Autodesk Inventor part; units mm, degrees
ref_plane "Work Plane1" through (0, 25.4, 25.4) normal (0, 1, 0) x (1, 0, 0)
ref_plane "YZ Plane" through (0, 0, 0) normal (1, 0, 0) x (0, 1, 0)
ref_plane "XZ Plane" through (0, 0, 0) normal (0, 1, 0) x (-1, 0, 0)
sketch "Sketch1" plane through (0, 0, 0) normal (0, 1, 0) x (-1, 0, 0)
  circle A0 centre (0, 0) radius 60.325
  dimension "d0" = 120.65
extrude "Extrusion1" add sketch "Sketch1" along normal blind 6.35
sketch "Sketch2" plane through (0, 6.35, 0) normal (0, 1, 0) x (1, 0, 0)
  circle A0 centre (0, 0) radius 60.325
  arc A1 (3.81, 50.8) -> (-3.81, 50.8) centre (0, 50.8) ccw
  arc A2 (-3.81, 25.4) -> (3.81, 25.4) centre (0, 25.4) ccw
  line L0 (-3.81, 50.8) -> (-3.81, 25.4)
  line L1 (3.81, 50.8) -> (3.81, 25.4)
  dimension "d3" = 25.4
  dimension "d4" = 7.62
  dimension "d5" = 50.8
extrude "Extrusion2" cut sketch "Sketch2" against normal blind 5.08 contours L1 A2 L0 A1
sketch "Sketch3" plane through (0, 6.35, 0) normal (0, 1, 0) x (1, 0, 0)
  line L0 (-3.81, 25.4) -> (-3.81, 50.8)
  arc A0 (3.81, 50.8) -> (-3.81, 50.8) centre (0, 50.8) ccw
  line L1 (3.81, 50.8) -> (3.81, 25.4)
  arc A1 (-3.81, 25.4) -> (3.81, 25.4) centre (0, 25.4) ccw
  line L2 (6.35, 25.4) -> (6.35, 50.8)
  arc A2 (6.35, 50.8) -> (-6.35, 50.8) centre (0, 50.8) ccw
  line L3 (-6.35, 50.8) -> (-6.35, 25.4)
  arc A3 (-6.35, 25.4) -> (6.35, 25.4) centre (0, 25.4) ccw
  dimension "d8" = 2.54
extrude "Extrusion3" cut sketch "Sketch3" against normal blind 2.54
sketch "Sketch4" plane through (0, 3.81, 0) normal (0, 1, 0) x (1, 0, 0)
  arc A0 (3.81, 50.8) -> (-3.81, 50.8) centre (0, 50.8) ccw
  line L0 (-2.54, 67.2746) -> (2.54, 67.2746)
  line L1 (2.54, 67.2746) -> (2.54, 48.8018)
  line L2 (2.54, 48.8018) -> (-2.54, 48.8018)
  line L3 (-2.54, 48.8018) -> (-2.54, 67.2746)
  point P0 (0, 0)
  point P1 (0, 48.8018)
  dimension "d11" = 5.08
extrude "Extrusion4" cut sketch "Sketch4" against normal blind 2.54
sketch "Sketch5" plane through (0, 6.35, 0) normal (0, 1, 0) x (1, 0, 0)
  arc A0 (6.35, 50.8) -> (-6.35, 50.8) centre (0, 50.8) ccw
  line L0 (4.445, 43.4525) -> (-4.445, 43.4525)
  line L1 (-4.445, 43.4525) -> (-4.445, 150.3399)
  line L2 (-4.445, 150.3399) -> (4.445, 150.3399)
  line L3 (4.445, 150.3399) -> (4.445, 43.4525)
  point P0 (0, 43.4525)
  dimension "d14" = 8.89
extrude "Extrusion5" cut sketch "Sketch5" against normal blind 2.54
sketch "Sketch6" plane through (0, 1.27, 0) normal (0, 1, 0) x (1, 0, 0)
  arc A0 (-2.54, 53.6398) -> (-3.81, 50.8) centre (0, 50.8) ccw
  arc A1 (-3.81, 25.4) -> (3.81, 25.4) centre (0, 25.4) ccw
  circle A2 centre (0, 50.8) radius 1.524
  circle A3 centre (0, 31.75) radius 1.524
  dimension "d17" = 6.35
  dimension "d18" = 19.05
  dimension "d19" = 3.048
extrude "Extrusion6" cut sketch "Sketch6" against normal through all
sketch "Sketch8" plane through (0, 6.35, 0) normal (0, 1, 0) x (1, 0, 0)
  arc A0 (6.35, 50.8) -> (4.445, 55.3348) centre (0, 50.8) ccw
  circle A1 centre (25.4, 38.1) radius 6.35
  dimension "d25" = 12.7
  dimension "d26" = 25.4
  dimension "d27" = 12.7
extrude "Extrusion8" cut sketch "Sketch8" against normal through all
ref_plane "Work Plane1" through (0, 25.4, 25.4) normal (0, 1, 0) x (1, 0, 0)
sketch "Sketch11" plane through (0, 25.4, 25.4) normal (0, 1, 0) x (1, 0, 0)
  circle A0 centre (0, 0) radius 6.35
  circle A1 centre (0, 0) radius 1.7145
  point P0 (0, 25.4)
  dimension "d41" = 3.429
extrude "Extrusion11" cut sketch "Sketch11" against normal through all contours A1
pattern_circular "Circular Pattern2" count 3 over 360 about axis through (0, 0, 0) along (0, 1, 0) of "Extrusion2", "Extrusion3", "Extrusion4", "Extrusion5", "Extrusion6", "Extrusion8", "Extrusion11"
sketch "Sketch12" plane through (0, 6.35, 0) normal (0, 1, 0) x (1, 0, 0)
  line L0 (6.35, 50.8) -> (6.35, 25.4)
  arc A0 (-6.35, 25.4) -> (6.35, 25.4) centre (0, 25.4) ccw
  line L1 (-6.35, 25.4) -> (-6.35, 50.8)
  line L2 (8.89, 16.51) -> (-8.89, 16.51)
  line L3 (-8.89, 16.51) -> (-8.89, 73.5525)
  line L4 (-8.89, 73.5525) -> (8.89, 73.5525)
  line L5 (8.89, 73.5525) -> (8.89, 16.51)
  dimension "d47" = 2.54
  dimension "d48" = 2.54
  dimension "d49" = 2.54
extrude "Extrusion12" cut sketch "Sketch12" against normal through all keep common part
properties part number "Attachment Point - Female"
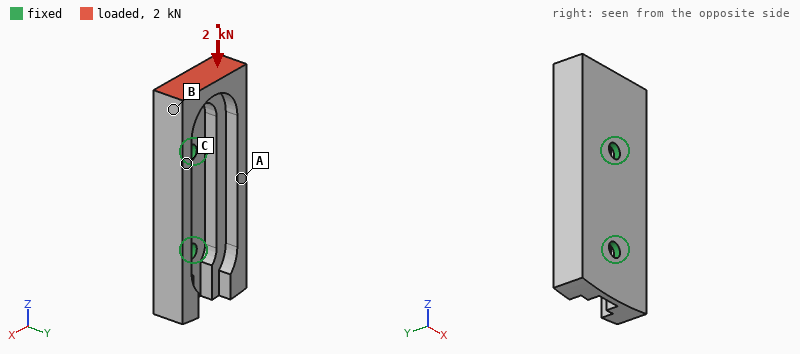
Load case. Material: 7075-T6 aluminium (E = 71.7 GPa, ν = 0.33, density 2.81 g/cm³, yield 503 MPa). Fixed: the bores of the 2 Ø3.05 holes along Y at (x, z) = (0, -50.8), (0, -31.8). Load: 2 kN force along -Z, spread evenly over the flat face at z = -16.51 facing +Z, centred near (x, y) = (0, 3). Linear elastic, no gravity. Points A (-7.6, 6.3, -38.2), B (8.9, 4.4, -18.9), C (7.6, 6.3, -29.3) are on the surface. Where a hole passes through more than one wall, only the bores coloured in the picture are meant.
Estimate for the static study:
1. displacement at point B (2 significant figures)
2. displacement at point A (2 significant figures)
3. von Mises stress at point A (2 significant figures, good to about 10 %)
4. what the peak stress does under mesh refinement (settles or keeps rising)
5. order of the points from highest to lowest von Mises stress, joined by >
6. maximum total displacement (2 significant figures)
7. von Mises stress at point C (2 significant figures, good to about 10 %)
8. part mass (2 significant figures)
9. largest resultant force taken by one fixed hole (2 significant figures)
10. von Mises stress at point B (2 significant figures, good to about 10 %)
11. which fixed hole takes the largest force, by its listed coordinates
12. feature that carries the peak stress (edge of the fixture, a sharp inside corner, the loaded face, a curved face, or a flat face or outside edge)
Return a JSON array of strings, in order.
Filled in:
["48 µm", "15 µm", "48 MPa", "keeps rising", "C > A > B", "68 µm", "74 MPa", "8.4 g", "1.2 kN", "24 MPa", "(0, -31.8)", "edge of the fixture"]
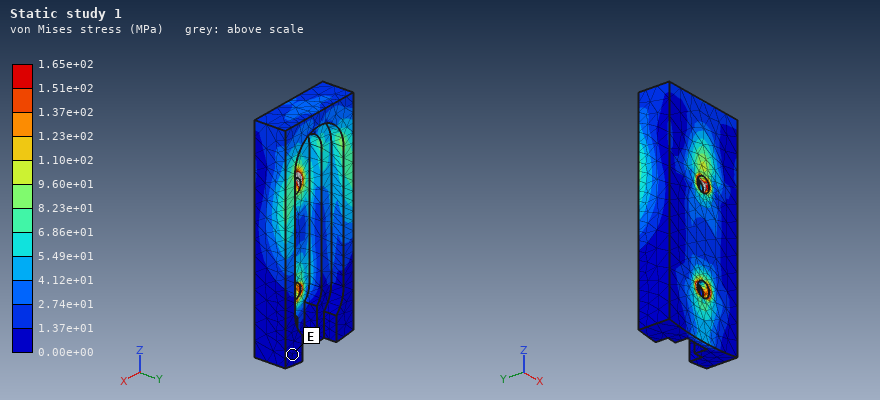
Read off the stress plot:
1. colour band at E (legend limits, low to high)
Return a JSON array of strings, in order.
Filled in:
["0.00e+00 to 1.37e+01 MPa"]
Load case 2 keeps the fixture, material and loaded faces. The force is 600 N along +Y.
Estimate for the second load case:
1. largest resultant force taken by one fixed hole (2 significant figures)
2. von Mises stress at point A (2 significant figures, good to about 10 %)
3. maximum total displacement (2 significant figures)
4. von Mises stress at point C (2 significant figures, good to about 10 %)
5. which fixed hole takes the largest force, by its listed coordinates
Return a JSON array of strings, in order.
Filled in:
["1.2 kN", "100 MPa", "0.18 mm", "140 MPa", "(0, -31.8)"]
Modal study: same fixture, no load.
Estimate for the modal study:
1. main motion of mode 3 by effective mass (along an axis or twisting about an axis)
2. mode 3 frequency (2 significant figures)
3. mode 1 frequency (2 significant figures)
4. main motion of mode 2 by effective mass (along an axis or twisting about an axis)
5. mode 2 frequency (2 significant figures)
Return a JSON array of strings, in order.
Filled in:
["along Y", "8600 Hz", "5100 Hz", "along Y", "7400 Hz"]
